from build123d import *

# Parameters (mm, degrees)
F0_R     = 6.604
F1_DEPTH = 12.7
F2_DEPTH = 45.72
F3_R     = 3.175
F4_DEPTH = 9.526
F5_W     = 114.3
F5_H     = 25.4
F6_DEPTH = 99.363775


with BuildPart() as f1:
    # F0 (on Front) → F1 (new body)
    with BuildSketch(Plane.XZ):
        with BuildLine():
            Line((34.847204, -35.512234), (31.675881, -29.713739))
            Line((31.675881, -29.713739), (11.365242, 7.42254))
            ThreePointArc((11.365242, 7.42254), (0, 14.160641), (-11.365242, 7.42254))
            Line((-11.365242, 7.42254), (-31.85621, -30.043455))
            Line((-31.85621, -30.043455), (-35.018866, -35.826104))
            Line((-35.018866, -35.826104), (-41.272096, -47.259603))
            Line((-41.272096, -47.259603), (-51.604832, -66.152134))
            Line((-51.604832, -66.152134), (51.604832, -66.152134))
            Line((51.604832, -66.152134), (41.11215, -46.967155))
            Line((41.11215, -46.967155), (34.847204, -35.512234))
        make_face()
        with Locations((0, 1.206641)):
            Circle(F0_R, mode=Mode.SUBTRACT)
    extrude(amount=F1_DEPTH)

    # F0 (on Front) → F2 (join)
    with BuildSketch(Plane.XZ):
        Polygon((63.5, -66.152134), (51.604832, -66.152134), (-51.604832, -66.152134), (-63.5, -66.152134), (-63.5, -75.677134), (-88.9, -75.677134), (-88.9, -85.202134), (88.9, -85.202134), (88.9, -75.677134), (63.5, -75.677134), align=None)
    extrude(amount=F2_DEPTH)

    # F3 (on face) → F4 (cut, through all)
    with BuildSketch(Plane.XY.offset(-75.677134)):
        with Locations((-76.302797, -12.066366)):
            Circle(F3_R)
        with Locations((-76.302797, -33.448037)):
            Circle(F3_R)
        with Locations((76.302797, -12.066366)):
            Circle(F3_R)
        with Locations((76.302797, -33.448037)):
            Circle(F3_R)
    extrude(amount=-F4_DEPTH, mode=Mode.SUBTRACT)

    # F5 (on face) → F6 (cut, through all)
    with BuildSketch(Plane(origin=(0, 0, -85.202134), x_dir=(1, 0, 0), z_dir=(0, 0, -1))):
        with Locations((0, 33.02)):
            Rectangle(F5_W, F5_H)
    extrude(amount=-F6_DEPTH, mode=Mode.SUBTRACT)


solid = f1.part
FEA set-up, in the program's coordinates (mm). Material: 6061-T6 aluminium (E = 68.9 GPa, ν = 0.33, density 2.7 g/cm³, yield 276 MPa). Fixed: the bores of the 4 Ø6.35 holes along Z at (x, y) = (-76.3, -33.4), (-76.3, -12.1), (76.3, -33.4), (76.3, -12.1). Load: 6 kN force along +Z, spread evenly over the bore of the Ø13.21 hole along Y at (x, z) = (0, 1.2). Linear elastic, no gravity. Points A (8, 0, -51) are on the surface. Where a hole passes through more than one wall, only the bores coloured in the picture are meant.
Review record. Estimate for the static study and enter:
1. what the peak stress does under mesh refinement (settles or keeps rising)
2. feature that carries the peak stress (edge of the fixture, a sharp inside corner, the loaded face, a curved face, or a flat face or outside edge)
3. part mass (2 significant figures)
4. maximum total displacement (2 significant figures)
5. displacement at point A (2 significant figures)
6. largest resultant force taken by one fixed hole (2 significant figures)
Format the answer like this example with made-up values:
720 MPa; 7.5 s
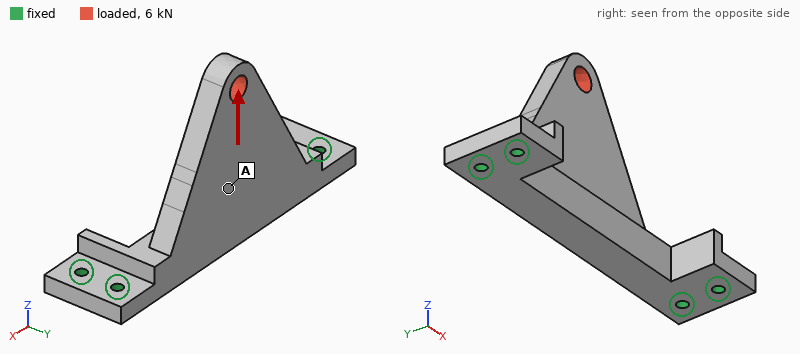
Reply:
keeps rising; edge of the fixture; 360 g; 0.16 mm; 0.082 mm; 4.4 kN
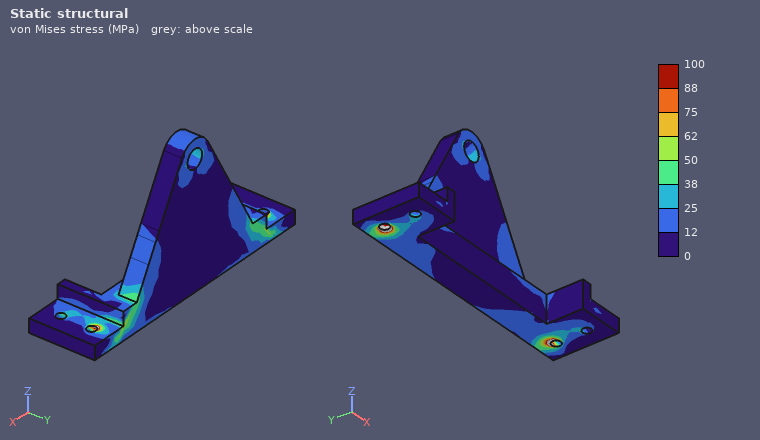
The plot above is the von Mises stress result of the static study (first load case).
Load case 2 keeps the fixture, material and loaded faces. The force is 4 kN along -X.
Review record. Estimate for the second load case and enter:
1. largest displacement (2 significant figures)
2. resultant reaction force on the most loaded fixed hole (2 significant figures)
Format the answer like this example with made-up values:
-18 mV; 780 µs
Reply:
87 µm; 2.9 kN
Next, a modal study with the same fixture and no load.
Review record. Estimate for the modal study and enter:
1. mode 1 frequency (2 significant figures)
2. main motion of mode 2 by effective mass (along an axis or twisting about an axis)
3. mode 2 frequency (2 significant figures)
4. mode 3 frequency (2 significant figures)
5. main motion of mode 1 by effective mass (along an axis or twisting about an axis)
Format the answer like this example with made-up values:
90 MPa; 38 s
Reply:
1200 Hz; along Z; 3400 Hz; 4300 Hz; along Y
